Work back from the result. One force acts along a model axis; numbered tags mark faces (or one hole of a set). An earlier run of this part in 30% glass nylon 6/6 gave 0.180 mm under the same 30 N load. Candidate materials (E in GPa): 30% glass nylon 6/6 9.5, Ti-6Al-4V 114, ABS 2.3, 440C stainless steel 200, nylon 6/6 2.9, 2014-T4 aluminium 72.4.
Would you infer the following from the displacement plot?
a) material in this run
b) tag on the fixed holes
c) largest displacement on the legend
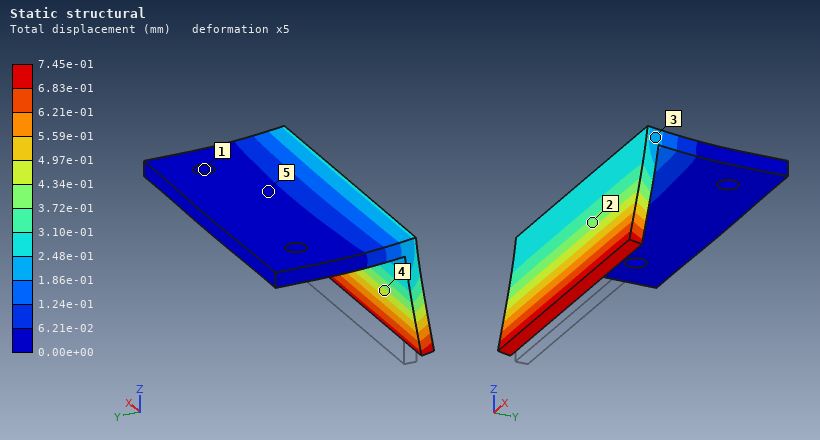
ABS
1
7.45e-01 mm
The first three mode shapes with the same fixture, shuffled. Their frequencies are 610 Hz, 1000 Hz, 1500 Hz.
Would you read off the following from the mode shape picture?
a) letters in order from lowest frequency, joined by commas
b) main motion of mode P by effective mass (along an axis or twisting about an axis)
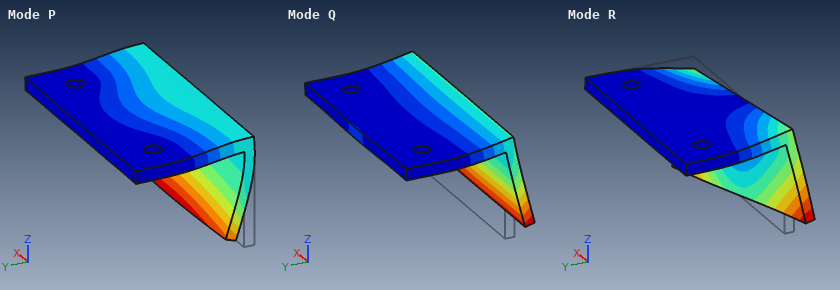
Q, R, P
along Z
